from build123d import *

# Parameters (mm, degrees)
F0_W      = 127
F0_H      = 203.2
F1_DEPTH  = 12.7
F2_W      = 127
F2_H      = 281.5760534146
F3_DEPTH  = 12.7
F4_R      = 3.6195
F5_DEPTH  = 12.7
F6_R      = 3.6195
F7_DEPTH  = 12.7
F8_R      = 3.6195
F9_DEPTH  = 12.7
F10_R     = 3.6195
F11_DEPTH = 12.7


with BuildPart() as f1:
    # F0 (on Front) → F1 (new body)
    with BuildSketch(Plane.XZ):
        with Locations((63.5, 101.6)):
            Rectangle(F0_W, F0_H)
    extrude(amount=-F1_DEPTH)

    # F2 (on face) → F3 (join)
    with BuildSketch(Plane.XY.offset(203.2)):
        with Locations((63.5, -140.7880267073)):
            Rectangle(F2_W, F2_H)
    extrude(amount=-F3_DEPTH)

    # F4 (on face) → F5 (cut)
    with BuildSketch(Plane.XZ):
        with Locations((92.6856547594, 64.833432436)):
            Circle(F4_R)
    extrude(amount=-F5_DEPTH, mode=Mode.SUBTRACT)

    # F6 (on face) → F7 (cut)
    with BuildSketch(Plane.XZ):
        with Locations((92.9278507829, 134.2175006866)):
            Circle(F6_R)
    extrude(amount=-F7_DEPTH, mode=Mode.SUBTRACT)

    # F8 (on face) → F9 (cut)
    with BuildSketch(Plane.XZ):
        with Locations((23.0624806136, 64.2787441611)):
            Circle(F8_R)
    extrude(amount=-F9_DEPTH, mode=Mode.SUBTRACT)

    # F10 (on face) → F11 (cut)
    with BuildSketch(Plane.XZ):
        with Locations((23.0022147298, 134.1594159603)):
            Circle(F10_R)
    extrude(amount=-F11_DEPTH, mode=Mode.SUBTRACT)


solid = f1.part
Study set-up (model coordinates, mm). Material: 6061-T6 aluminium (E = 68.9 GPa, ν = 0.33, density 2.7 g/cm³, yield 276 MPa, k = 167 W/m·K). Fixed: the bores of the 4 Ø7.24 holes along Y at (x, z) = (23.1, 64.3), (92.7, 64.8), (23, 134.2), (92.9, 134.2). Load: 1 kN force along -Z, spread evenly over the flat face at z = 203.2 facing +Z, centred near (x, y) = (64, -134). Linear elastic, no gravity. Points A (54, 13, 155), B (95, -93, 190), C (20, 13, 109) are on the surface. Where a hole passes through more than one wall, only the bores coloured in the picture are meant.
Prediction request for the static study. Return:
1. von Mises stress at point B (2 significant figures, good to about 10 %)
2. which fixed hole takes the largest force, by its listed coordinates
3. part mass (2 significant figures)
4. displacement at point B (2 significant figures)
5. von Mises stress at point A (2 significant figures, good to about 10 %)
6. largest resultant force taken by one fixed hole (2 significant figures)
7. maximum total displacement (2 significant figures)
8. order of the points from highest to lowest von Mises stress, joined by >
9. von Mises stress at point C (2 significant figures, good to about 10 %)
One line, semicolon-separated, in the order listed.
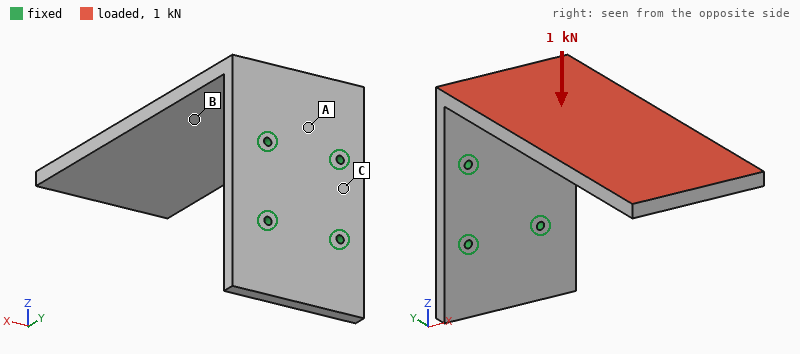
17 MPa; (92.9, 134.2); 2.1 kg; 0.90 mm; 34 MPa; 720 N; 3.4 mm; A > B > C; 6.2 MPa
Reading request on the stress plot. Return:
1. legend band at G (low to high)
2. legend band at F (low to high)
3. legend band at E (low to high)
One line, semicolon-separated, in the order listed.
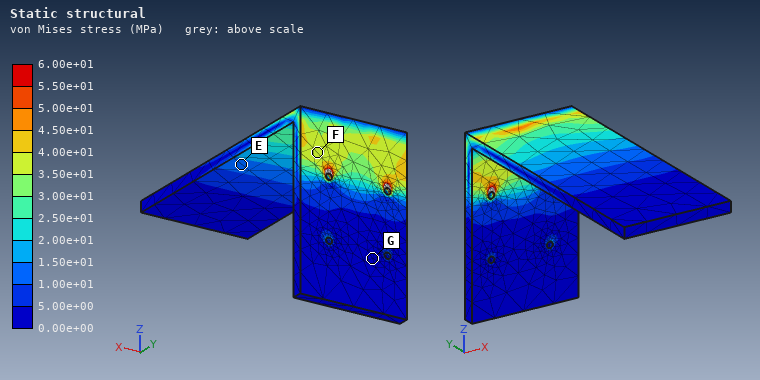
0.00e+00 to 5.00e+00 MPa; 3.50e+01 to 4.00e+01 MPa; 1.00e+01 to 1.50e+01 MPa
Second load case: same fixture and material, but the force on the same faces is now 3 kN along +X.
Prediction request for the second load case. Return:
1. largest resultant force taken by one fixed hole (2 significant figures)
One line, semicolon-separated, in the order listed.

6.3 kN
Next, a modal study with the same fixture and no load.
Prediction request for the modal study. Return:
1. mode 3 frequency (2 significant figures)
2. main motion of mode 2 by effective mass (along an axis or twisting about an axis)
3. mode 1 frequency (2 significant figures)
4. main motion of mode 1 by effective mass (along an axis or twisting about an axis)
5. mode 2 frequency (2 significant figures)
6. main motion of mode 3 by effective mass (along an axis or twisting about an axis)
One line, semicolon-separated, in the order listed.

540 Hz; along X; 94 Hz; along Z; 220 Hz; along Y
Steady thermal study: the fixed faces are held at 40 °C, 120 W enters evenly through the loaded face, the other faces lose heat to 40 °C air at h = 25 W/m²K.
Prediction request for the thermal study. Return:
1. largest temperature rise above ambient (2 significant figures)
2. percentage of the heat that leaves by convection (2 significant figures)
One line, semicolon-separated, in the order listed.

51 K; 43 %
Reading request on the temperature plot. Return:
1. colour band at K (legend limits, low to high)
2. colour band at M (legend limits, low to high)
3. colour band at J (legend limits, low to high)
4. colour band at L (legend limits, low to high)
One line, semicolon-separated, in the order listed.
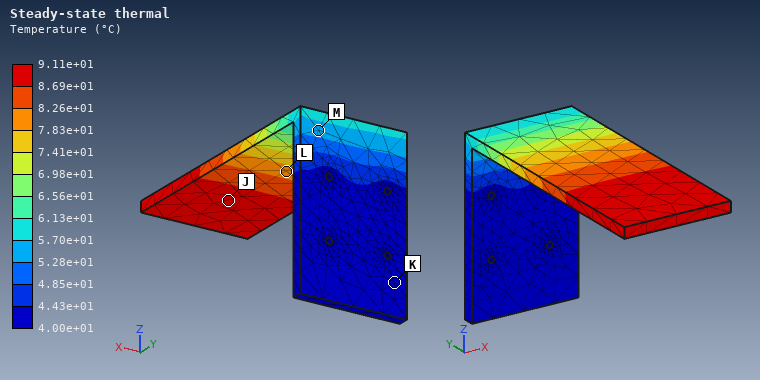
4.00e+01 to 4.43e+01 °C; 5.28e+01 to 5.70e+01 °C; 8.69e+01 to 9.11e+01 °C; 7.83e+01 to 8.26e+01 °C
